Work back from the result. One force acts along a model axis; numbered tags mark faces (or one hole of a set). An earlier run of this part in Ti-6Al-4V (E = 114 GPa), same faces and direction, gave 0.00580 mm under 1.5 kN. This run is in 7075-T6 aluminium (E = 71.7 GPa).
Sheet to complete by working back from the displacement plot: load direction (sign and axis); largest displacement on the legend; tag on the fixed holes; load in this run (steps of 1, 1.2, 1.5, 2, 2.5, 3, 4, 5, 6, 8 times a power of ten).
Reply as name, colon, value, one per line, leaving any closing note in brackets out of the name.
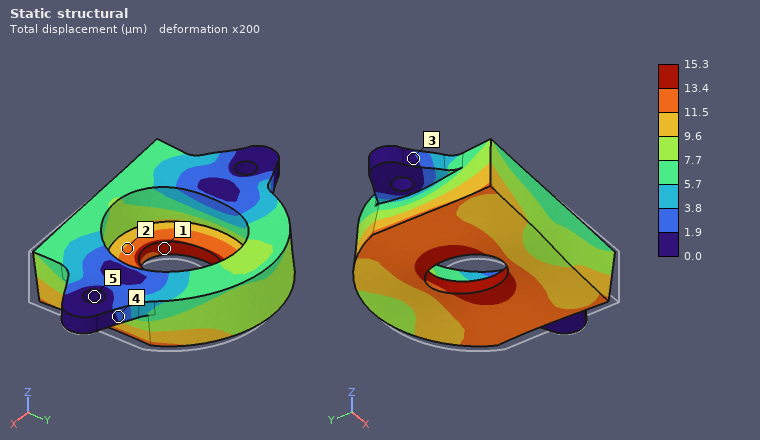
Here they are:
load direction: -X
largest displacement on the legend: 15.3 µm
tag on the fixed holes: 5
load in this run: 2.5 kN
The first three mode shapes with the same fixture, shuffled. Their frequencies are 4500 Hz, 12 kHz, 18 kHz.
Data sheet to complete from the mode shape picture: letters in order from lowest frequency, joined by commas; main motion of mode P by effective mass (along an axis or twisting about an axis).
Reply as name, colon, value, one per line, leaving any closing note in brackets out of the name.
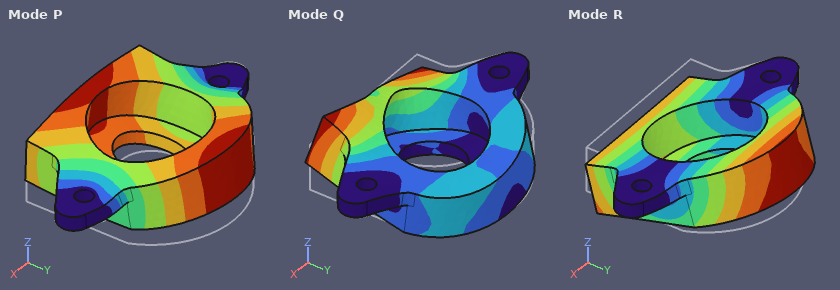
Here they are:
letters in order from lowest frequency, joined by commas: R, P, Q
main motion of mode P by effective mass: along Z
